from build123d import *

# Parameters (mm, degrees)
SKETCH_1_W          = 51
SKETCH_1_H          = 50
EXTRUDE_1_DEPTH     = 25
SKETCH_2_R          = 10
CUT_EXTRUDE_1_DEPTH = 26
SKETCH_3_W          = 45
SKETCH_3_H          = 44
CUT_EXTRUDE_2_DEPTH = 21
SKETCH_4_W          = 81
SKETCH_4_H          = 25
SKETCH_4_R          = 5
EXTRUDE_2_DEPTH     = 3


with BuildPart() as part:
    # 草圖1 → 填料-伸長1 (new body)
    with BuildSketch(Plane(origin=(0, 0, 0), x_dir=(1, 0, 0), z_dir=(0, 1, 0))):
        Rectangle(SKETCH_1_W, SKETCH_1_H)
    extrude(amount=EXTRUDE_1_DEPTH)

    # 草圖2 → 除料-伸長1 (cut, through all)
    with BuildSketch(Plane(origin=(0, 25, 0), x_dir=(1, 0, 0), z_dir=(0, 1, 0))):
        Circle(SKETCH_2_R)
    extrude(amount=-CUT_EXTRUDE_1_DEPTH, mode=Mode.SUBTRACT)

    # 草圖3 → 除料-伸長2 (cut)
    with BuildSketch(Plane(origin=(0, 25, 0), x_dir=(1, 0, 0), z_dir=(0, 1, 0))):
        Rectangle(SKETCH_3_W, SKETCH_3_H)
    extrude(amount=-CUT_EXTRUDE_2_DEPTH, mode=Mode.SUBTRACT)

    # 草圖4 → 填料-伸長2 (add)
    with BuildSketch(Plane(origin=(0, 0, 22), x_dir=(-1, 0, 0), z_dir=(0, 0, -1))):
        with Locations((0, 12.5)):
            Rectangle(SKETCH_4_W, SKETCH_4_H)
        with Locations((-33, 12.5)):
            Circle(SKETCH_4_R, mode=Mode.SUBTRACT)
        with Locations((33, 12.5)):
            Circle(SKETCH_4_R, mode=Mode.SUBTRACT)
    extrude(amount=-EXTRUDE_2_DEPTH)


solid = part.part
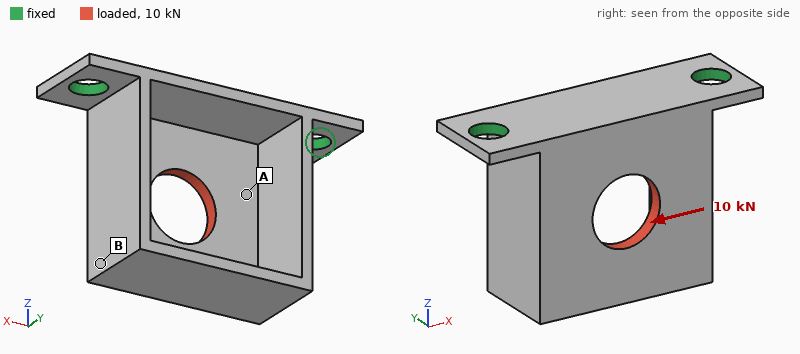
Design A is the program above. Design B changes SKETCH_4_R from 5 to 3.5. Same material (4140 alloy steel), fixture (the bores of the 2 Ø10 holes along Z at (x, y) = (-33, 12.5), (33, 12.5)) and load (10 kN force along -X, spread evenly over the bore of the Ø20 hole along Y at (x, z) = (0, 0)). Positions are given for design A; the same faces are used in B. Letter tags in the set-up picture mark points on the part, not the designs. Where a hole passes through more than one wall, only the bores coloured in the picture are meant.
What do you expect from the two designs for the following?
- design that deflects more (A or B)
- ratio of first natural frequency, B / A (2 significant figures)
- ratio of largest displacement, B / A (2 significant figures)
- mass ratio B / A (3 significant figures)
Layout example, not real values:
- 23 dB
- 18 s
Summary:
- B
- 0.78
- 1.2
- 1.01
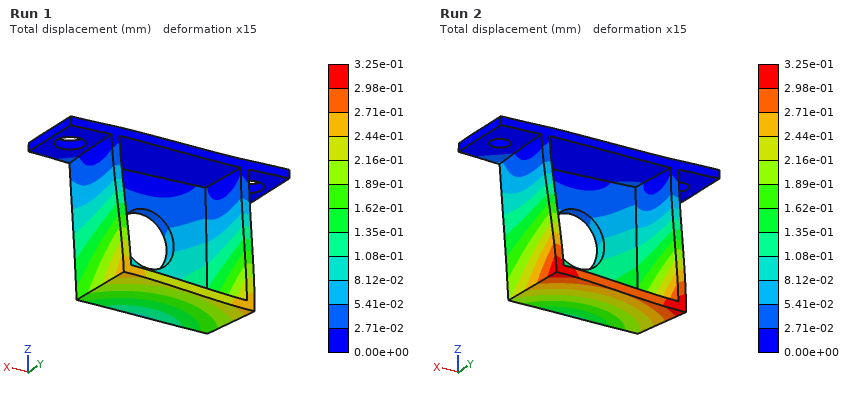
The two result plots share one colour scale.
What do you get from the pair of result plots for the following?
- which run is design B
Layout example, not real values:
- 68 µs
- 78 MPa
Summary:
- Run 2
